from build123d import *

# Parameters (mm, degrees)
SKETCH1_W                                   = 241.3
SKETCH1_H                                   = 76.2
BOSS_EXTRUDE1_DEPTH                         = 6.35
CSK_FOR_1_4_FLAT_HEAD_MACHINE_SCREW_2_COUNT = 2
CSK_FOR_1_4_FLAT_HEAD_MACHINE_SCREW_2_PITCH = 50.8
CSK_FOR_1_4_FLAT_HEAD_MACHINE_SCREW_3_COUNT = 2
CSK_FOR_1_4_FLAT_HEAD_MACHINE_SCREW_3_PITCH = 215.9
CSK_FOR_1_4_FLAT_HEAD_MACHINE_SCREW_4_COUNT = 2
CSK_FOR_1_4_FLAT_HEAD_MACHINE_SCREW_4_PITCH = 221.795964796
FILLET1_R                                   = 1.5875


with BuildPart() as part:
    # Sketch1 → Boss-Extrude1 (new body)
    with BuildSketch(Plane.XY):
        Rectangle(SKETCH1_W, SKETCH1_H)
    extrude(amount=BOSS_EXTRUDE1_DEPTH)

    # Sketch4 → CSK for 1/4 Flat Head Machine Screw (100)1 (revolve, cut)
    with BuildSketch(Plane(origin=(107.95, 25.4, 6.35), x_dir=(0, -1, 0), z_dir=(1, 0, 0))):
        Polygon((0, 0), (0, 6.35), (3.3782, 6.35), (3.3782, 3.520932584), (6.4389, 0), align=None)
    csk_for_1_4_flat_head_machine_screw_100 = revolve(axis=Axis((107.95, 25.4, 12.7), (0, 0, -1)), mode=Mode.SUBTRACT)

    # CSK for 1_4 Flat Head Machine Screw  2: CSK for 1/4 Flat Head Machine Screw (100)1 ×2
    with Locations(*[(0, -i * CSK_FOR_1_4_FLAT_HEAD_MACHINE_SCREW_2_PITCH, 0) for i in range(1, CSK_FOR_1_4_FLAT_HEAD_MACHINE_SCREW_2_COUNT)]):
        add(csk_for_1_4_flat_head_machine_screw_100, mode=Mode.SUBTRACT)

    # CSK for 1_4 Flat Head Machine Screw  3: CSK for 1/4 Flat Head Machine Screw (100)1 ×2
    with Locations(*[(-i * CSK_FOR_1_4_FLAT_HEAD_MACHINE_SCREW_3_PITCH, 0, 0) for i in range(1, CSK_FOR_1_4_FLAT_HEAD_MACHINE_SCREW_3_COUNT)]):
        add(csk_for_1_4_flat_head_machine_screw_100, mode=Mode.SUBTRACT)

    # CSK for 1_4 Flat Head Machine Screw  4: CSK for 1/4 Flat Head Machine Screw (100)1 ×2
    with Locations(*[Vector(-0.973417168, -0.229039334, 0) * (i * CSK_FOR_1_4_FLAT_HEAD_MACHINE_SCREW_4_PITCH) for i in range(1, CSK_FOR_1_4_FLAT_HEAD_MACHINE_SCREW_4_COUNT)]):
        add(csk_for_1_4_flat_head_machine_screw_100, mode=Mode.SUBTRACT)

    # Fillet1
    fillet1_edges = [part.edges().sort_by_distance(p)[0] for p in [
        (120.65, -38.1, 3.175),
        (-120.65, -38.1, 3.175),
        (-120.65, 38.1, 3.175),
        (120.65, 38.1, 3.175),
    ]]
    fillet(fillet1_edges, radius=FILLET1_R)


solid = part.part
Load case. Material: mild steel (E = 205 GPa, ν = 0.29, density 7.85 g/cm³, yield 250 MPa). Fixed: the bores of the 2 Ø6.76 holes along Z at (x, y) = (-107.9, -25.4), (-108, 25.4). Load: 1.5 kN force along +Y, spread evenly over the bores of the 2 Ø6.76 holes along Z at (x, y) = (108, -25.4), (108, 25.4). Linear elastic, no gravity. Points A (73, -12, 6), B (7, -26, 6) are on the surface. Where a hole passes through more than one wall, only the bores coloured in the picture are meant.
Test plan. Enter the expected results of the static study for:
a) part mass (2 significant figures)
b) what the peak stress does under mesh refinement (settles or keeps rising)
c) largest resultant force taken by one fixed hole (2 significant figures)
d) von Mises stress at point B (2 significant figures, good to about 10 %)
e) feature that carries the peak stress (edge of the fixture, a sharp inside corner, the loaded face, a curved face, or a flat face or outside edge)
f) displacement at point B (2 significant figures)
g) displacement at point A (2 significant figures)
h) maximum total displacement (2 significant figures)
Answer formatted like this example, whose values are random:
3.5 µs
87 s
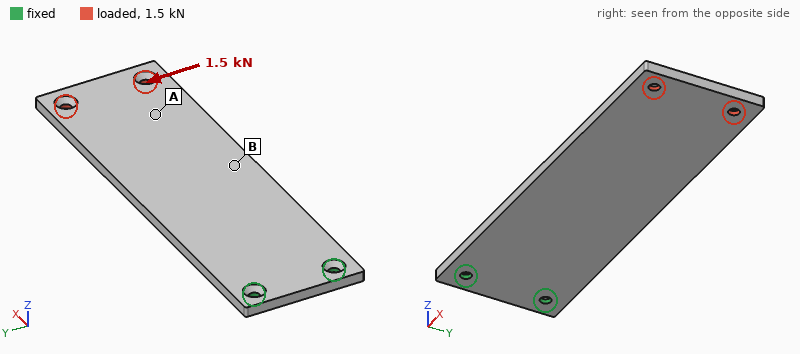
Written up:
900 g
keeps rising
6.1 kN
17 MPa
edge of the fixture
0.059 mm
0.10 mm
0.16 mm
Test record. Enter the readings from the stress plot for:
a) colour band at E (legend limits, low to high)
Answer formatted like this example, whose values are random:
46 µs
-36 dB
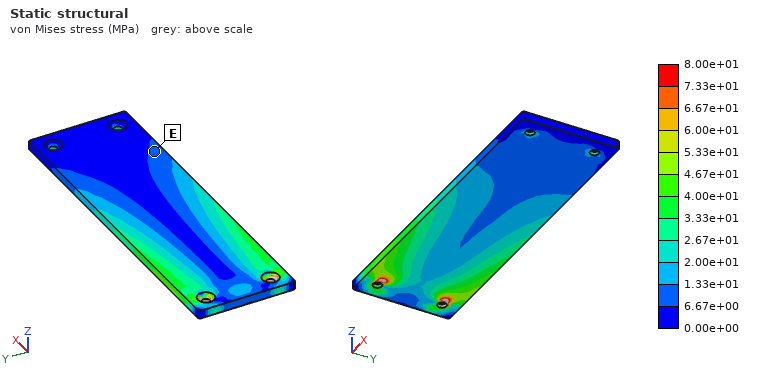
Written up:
6.67e+00 to 1.33e+01 MPa
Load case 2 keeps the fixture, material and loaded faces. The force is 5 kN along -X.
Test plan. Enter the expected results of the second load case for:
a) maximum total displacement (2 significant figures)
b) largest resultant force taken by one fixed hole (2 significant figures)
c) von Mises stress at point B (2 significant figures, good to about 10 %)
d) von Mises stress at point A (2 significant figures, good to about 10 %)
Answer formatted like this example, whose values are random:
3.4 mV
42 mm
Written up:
0.68 mm
2.5 kN
6.9 MPa
7.9 MPa
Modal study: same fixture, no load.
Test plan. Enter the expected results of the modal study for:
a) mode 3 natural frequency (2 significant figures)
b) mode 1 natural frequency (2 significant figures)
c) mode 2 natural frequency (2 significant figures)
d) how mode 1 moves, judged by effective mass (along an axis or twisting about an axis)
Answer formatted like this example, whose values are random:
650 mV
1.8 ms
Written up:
610 Hz
93 Hz
590 Hz
along Z
